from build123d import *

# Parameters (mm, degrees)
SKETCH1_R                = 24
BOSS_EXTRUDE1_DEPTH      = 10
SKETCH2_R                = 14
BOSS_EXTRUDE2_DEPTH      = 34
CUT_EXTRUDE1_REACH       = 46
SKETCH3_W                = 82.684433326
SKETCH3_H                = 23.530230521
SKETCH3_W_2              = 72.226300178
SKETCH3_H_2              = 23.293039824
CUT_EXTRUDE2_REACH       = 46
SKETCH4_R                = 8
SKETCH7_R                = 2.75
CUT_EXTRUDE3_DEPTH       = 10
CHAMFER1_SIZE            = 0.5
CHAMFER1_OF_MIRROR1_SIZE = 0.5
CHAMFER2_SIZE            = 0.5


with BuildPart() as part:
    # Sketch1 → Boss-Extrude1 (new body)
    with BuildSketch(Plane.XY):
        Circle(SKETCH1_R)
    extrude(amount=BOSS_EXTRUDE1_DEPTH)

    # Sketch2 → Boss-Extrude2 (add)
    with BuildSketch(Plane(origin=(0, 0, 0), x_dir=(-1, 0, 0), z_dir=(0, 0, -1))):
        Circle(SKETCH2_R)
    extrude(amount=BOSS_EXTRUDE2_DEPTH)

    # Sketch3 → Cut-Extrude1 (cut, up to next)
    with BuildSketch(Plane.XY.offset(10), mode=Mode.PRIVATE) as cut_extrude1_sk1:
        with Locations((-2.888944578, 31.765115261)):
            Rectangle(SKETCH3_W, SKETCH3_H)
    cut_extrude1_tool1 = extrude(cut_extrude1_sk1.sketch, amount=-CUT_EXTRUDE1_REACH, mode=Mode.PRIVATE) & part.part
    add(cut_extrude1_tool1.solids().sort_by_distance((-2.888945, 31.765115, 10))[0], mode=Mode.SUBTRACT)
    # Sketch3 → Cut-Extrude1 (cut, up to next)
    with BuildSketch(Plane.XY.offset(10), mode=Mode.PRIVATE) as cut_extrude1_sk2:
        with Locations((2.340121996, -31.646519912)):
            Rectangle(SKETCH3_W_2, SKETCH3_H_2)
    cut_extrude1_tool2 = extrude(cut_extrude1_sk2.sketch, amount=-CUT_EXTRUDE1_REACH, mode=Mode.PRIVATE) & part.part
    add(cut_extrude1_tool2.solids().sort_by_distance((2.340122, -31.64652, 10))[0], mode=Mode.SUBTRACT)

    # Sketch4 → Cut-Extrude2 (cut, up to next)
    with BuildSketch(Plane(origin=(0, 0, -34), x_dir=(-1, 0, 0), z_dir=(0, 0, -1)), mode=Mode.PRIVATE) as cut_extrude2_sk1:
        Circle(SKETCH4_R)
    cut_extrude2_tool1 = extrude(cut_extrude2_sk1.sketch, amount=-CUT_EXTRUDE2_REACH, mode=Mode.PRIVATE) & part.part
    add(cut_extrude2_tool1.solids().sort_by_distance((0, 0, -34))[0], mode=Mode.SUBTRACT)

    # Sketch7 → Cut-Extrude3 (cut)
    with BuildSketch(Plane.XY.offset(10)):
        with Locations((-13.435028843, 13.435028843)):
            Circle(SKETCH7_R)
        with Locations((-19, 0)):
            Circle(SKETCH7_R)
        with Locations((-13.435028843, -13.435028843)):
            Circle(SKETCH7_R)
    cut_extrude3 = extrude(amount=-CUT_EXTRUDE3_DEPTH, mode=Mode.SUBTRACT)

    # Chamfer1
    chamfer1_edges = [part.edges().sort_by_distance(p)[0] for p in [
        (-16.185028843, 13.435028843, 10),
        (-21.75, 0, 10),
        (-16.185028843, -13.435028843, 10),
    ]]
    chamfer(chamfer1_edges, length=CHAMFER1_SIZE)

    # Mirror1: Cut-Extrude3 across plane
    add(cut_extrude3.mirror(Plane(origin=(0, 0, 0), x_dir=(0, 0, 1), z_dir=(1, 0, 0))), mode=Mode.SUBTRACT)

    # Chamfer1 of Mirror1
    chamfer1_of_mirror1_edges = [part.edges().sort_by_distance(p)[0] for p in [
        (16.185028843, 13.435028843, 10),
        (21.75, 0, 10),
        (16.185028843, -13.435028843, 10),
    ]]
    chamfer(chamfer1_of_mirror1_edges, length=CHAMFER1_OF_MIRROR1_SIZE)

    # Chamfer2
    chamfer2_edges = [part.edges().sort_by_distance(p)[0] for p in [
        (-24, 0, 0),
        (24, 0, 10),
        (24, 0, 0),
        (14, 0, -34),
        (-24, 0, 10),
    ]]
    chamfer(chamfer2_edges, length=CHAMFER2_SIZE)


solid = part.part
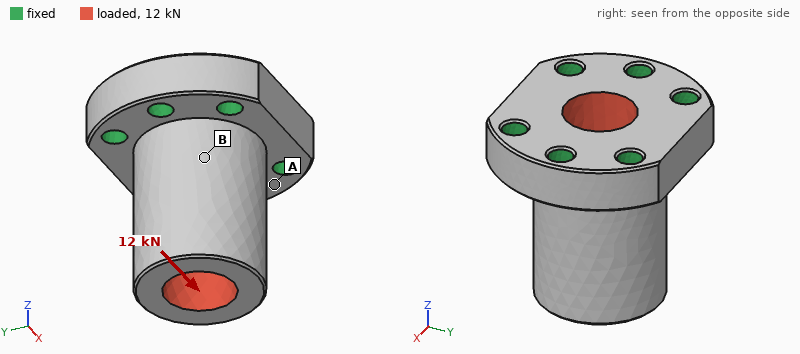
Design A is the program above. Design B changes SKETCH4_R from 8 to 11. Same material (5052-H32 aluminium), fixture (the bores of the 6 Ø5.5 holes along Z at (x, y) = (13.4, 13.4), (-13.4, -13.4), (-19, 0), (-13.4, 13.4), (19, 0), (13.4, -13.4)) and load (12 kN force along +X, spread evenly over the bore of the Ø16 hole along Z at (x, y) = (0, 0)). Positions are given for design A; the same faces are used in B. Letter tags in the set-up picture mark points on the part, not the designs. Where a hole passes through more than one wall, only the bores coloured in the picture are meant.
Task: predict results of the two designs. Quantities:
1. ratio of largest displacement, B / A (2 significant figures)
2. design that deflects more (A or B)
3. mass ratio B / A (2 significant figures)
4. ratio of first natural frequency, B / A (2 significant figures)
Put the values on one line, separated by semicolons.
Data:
1.6; B; 0.71; 1.1
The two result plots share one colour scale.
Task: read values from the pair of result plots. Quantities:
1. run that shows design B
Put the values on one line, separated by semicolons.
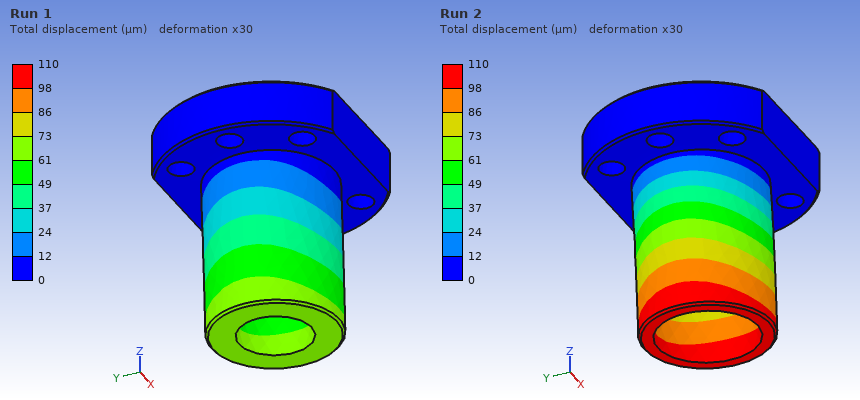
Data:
Run 2
